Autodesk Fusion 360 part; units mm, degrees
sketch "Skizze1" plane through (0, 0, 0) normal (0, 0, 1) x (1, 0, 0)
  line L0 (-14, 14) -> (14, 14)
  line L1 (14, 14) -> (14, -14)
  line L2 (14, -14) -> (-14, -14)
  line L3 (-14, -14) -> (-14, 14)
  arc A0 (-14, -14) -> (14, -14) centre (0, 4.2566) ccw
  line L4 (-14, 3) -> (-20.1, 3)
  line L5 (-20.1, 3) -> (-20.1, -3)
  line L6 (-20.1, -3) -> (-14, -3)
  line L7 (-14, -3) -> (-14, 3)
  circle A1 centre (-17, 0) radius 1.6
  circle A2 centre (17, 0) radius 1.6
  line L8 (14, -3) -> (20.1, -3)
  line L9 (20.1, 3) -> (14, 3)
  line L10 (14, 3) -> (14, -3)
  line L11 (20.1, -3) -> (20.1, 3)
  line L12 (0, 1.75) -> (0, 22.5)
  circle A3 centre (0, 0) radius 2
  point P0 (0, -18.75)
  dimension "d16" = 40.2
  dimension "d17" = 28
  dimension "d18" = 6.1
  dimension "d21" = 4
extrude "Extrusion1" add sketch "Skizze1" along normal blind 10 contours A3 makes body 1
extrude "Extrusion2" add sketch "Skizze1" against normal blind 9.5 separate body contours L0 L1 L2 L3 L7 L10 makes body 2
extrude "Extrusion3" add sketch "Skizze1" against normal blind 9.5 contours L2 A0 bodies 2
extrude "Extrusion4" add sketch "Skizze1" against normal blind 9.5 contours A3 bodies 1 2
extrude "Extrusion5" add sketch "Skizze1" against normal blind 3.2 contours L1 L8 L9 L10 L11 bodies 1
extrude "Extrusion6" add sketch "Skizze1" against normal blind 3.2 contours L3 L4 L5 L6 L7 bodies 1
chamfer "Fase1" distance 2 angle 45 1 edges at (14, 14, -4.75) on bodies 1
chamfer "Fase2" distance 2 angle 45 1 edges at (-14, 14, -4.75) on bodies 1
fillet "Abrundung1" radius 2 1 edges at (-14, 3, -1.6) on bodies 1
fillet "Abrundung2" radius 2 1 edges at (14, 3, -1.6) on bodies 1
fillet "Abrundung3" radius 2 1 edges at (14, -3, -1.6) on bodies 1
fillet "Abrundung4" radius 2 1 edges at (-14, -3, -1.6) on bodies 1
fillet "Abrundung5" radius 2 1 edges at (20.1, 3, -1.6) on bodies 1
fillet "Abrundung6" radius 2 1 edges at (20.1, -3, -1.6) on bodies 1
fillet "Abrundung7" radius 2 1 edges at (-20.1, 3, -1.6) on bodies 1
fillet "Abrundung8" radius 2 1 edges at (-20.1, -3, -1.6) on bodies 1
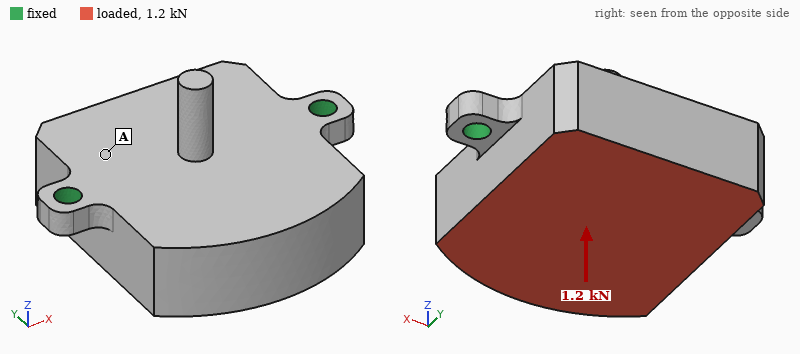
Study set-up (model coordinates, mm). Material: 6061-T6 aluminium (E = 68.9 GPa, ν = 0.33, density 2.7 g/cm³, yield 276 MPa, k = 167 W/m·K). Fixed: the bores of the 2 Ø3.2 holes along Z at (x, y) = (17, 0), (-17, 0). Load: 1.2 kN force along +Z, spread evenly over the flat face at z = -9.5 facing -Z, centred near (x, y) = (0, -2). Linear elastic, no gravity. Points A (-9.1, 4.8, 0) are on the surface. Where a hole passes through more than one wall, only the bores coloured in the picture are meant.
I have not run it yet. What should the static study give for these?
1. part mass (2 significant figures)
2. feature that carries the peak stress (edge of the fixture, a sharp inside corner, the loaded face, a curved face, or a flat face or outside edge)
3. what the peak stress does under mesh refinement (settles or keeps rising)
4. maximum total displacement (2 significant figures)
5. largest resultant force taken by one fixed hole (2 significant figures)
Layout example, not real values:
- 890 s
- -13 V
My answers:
- 23 g
- edge of the fixture
- keeps rising
- 50 µm
- 700 N
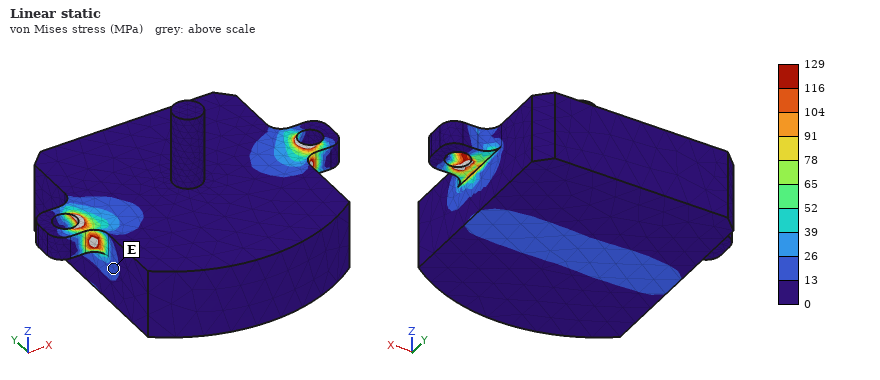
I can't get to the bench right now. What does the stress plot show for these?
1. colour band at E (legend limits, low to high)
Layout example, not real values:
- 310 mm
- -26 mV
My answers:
- 13 to 26 MPa
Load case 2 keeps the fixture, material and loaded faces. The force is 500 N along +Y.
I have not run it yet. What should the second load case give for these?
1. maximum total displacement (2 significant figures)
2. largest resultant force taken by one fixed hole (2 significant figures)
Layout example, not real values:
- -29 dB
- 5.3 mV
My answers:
- 74 µm
- 250 N
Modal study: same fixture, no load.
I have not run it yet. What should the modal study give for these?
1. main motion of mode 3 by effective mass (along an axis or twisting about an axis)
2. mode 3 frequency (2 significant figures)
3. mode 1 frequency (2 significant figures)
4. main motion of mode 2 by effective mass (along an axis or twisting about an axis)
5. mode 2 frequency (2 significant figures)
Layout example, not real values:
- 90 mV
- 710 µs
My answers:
- along Y
- 18 kHz
- 3500 Hz
- along Z
- 12 kHz
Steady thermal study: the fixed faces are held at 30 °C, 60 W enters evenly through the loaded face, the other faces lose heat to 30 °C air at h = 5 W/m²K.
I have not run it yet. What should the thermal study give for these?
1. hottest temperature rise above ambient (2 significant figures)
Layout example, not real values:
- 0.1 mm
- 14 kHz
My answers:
- 41 K
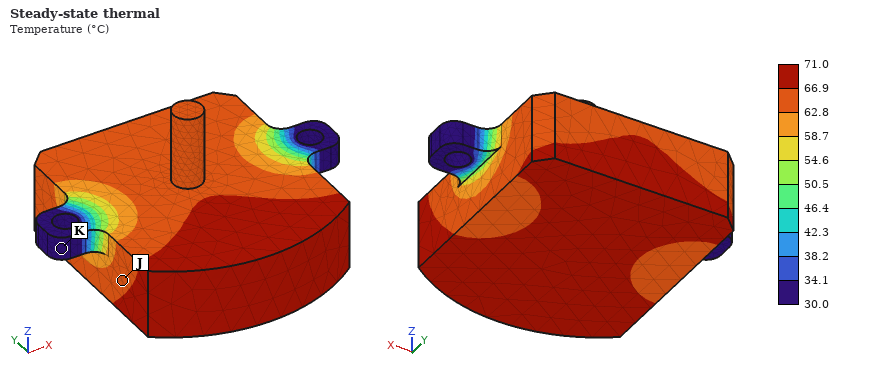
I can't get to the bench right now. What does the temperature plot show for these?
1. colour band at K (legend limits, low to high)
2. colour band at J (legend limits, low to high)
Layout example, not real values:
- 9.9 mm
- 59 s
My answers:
- 30.0 to 34.1 °C
- 62.8 to 66.9 °C
